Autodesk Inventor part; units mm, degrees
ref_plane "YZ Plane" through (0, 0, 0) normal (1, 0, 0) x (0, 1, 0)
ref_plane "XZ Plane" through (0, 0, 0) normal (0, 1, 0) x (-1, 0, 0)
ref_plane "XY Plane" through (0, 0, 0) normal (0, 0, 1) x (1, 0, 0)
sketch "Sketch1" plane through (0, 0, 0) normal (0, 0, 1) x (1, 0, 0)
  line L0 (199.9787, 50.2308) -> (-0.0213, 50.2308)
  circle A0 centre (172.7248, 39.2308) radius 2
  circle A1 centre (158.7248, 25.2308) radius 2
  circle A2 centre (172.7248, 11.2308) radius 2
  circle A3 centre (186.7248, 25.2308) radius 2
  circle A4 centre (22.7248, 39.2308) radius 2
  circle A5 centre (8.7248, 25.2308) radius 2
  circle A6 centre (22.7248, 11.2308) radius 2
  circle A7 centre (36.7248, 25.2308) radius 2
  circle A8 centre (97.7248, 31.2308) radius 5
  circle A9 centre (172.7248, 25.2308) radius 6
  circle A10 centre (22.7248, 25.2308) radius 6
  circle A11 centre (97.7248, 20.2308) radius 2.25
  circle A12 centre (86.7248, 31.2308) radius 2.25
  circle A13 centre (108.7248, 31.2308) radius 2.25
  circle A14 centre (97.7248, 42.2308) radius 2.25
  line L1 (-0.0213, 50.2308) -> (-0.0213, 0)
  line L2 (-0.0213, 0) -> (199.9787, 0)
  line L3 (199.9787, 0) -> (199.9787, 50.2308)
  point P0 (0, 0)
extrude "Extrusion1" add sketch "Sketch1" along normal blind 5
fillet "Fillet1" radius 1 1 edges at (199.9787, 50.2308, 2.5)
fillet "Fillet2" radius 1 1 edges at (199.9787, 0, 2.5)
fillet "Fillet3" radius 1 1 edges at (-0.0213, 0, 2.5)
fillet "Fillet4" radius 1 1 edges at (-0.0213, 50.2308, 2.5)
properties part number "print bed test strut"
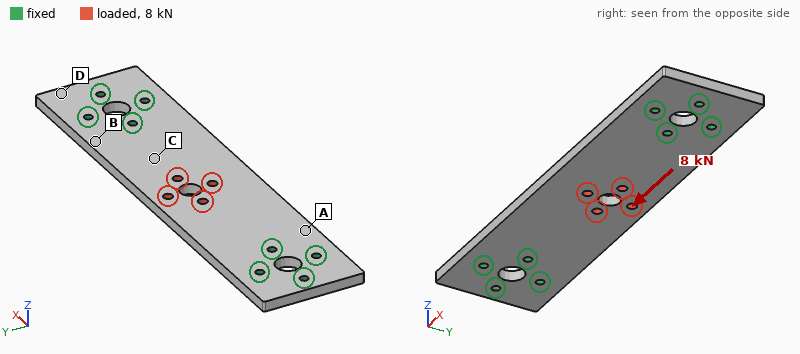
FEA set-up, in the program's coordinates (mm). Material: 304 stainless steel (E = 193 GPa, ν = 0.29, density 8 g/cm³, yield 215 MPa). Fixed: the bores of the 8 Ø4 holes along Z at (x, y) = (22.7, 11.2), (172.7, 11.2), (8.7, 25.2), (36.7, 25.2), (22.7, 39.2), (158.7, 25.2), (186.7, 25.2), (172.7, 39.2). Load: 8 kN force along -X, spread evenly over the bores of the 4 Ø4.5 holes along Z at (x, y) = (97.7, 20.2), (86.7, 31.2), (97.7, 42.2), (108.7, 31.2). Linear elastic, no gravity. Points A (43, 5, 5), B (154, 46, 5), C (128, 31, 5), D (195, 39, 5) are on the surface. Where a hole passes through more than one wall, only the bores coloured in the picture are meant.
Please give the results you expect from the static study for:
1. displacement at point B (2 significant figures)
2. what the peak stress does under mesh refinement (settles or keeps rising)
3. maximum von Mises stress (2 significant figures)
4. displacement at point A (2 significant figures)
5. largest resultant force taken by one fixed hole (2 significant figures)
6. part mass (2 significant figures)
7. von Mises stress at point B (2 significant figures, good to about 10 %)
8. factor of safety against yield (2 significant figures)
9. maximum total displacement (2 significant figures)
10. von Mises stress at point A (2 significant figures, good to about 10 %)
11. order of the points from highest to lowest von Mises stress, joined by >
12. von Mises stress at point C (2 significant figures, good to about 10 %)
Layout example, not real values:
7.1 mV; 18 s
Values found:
1.7 µm; settles; 69 MPa; 1.7 µm; 1.9 kN; 380 g; 14 MPa; 3.1; 7.1 µm; 11 MPa; C > B > A > D; 22 MPa
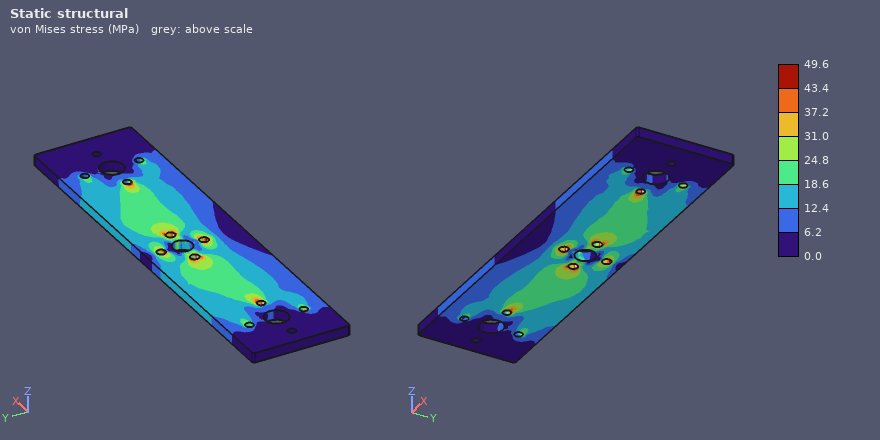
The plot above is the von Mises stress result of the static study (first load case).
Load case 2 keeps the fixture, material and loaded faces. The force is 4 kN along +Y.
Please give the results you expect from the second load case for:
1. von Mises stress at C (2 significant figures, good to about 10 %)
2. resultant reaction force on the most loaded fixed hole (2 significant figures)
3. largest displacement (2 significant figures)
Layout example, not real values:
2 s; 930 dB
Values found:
19 MPa; 2.2 kN; 15 µm
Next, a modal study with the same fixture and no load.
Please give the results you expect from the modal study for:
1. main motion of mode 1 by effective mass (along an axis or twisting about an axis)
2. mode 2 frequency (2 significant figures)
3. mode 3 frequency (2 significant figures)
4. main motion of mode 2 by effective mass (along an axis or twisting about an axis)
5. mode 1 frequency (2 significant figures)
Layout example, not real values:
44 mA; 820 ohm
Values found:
along Z; 2500 Hz; 4000 Hz; twisting about X; 1500 Hz
